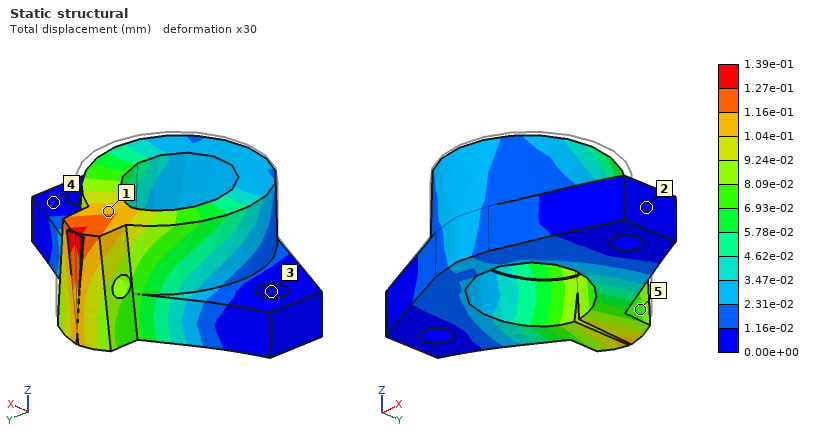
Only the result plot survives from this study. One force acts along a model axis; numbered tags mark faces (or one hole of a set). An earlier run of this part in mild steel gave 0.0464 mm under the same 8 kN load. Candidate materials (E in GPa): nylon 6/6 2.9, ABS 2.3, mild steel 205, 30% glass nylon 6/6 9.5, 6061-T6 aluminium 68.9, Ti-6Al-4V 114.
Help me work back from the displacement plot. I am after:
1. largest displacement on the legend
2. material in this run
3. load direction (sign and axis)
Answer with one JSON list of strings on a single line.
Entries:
["1.39e-01 mm", "6061-T6 aluminium", "-Z"]
